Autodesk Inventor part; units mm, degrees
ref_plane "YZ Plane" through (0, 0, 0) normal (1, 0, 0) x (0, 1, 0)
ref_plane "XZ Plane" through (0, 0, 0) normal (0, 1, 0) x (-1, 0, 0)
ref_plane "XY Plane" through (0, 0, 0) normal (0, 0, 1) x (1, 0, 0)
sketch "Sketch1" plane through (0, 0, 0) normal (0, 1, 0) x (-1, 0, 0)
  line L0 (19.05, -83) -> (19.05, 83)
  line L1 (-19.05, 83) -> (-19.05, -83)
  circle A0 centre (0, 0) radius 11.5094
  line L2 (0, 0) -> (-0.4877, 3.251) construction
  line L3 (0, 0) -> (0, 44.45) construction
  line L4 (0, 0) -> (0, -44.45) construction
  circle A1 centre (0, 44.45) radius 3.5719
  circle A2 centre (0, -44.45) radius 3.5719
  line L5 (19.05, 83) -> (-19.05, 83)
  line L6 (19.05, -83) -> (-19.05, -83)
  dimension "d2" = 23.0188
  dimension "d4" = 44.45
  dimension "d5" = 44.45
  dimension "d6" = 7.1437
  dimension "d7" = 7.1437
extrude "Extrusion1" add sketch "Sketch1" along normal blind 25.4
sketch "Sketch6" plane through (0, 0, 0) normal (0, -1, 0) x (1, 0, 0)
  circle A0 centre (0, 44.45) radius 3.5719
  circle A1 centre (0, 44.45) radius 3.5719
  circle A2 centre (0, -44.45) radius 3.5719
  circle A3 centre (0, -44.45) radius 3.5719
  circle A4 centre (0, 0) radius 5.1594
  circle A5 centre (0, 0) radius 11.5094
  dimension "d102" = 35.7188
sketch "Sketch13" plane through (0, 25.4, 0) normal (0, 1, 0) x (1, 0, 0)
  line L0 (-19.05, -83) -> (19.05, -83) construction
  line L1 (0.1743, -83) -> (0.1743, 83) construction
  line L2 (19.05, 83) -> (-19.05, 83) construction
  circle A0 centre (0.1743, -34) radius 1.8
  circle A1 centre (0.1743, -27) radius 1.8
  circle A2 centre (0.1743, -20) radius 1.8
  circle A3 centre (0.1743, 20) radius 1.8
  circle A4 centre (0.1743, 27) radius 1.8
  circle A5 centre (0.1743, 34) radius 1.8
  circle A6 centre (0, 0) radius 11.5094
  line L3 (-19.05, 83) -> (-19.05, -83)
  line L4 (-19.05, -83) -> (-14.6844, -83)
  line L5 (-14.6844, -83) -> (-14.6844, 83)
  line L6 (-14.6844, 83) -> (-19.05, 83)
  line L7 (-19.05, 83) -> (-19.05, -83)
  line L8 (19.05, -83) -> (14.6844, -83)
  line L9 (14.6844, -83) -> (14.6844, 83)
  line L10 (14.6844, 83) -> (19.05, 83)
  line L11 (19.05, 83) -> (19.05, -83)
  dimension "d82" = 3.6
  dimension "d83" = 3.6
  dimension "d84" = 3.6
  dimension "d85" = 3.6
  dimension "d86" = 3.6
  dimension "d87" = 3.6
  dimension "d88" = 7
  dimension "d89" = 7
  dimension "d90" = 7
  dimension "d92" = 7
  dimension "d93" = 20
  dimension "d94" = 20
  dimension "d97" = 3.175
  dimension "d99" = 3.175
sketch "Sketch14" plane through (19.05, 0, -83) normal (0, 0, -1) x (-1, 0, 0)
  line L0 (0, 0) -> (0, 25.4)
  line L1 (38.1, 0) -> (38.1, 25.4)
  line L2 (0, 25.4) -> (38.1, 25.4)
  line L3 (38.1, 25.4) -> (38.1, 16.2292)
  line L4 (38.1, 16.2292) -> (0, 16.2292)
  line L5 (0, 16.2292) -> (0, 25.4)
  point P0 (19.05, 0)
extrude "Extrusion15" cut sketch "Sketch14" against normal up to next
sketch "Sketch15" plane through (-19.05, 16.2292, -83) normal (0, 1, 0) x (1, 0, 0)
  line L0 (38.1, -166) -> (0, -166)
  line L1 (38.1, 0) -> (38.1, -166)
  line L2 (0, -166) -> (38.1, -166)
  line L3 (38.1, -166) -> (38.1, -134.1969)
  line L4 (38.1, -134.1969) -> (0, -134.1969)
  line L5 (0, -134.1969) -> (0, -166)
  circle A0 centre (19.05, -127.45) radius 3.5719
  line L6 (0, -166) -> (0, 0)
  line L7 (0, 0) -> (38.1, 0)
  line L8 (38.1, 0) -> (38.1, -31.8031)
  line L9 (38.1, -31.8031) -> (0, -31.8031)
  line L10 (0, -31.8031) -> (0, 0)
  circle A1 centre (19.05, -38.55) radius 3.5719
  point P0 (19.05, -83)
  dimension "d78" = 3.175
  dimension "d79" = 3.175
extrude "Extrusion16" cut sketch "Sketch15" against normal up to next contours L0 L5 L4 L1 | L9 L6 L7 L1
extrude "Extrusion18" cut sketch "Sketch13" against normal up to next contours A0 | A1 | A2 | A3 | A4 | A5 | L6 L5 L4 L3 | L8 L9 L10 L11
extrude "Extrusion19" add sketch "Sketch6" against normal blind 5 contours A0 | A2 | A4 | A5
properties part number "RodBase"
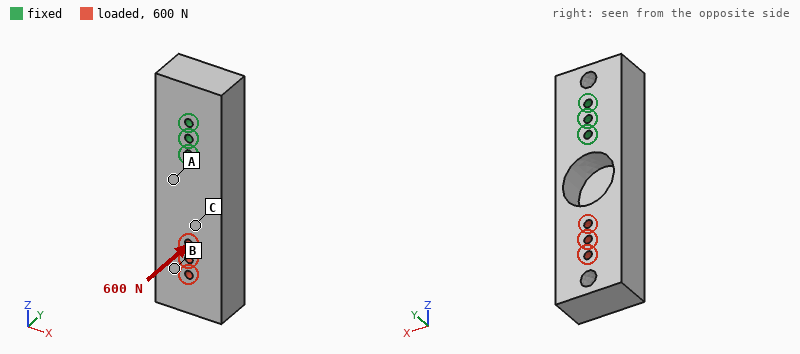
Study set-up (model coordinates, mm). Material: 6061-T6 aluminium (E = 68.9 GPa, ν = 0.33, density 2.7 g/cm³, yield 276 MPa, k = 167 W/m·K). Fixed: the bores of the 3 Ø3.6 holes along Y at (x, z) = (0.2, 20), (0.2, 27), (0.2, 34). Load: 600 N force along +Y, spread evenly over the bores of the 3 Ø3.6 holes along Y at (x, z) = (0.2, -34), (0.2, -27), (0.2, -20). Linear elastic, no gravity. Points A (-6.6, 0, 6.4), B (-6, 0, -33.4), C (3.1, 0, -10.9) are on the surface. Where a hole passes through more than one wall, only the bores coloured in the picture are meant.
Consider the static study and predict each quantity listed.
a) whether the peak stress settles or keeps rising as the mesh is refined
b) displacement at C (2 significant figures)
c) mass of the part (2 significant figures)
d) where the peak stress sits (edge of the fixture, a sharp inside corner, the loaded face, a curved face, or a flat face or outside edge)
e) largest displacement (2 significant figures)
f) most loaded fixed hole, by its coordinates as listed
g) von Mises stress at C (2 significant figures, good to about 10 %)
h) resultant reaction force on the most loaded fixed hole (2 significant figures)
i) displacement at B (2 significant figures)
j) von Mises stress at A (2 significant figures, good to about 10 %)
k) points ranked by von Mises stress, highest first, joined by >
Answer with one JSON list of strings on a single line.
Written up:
["keeps rising", "0.037 mm", "110 g", "edge of the fixture", "0.11 mm", "(0.2, 20)", "10 MPa", "1.2 kN", "0.079 mm", "22 MPa", "A > C > B"]
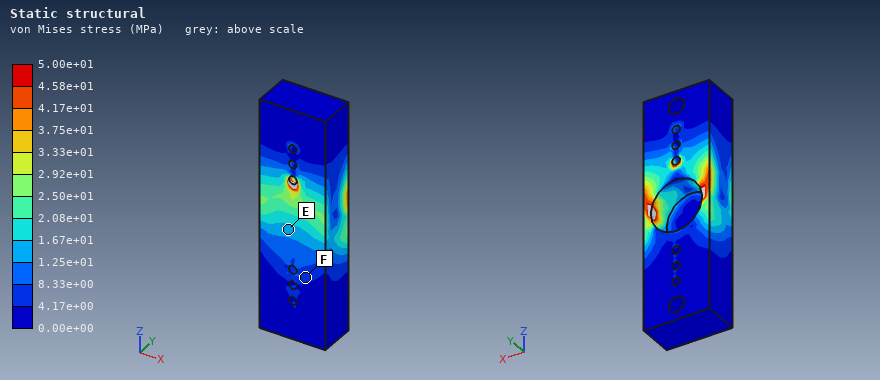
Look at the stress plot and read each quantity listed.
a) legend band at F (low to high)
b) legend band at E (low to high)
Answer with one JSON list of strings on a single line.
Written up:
["4.17e+00 to 8.33e+00 MPa", "1.25e+01 to 1.67e+01 MPa"]
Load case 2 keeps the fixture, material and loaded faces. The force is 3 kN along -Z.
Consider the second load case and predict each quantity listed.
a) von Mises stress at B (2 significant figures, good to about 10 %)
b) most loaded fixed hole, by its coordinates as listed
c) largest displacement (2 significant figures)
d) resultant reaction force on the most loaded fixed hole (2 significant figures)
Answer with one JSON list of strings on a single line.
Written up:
["3.4 MPa", "(0.2, 20)", "43 µm", "1.5 kN"]
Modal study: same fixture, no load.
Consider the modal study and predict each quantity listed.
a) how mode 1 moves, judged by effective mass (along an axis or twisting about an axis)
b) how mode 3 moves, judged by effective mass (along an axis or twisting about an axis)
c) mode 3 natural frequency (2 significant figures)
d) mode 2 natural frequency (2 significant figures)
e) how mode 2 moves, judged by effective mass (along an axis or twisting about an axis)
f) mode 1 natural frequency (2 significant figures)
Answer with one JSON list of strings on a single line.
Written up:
["along Y", "twisting about Z", "6200 Hz", "2800 Hz", "along X", "1800 Hz"]
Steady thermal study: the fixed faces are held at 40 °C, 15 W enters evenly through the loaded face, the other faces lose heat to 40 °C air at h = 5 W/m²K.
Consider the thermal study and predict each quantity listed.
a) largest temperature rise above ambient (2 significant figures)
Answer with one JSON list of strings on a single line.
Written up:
["14 K"]
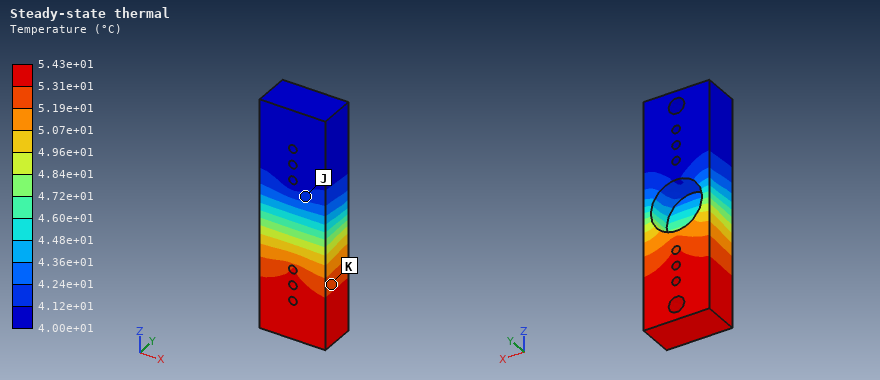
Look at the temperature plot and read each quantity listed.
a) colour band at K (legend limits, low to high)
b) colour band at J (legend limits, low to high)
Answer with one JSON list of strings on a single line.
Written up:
["5.19e+01 to 5.31e+01 °C", "4.12e+01 to 4.24e+01 °C"]
